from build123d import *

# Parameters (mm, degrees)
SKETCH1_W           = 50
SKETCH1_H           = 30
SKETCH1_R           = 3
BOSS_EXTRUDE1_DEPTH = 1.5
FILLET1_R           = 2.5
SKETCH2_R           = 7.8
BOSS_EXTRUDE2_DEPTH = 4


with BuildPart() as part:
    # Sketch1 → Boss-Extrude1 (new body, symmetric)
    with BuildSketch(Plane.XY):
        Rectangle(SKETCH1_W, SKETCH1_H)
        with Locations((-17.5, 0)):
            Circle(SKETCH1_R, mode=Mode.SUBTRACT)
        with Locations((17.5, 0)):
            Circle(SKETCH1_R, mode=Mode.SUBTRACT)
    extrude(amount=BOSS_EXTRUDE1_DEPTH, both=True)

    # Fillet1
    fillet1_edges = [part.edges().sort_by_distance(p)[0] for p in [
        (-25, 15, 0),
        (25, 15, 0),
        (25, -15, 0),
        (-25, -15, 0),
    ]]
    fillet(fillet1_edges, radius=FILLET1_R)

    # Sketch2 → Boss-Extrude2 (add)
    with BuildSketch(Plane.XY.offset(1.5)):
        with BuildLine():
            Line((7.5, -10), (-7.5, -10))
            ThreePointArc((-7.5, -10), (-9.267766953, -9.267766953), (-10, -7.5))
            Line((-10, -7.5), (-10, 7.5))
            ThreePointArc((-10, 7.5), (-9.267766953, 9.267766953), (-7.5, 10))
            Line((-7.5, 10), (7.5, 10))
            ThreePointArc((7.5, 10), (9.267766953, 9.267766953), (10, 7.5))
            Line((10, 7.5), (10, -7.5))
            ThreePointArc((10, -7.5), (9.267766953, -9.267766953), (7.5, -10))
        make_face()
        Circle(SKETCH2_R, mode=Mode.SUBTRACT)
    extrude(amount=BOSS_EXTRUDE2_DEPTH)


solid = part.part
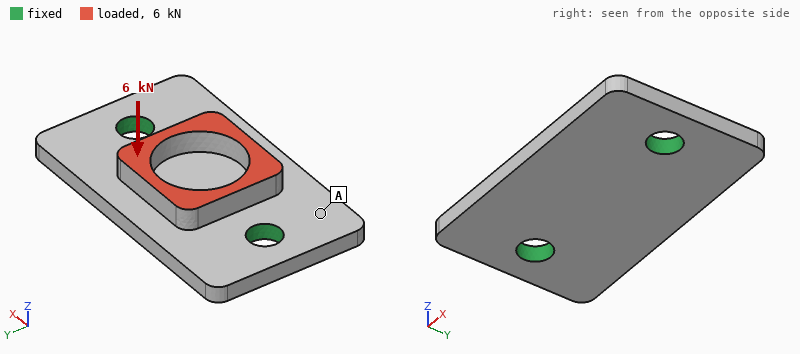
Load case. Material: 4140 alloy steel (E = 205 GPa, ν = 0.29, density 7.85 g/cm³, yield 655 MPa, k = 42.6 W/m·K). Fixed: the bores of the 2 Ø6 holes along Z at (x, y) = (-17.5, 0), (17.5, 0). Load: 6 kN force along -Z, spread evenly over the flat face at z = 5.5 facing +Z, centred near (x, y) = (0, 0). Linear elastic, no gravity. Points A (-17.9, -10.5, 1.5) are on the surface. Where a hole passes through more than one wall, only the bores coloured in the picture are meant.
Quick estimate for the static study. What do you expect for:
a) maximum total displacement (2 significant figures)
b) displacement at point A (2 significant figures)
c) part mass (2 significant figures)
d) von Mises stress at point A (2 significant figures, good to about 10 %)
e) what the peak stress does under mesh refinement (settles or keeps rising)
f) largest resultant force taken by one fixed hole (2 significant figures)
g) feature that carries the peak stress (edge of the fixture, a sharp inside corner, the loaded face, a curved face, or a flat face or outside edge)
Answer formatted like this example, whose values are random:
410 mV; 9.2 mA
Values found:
50 µm; 9.5 µm; 40 g; 63 MPa; keeps rising; 3.2 kN; edge of the fixture
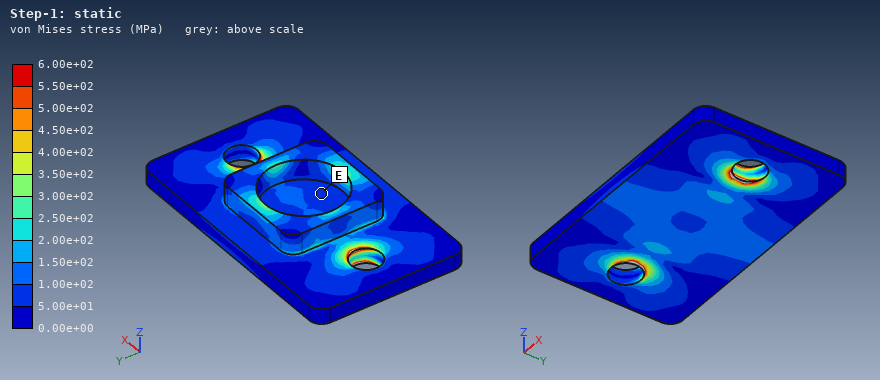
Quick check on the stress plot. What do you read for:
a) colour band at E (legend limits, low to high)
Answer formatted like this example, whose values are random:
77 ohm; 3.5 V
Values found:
5.00e+01 to 1.00e+02 MPa
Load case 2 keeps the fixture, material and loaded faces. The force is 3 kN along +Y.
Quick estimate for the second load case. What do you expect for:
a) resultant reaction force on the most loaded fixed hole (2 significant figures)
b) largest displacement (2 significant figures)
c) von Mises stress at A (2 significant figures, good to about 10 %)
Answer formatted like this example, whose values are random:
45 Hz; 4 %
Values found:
1.5 kN; 40 µm; 51 MPa
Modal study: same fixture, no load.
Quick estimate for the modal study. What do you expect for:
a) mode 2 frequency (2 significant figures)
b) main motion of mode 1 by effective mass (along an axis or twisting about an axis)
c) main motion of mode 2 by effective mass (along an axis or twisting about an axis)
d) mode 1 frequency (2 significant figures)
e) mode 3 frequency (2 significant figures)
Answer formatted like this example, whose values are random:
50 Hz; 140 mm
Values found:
13 kHz; twisting about X; along Z; 9300 Hz; 16 kHz
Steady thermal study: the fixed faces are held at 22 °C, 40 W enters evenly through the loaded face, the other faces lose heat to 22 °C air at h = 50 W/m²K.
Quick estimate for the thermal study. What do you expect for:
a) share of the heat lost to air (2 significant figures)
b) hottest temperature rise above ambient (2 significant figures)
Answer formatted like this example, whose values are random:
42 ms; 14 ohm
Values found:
16 %; 75 K
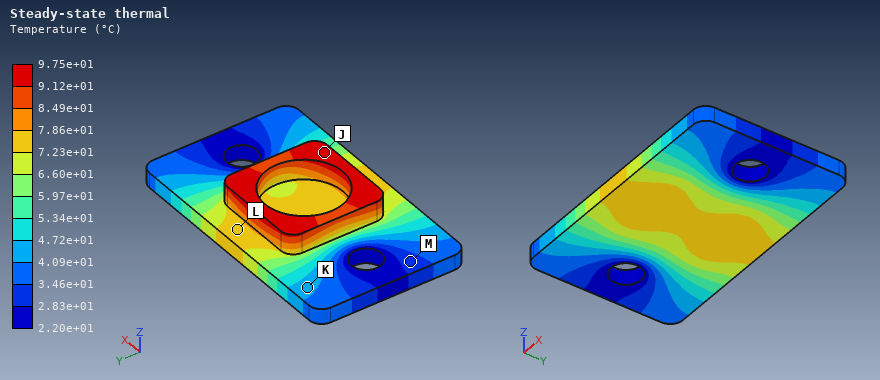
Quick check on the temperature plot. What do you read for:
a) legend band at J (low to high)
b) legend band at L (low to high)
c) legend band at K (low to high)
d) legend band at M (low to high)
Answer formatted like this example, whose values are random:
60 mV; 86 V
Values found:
9.12e+01 to 9.75e+01 °C; 7.23e+01 to 7.86e+01 °C; 4.09e+01 to 4.72e+01 °C; 2.83e+01 to 3.46e+01 °C
